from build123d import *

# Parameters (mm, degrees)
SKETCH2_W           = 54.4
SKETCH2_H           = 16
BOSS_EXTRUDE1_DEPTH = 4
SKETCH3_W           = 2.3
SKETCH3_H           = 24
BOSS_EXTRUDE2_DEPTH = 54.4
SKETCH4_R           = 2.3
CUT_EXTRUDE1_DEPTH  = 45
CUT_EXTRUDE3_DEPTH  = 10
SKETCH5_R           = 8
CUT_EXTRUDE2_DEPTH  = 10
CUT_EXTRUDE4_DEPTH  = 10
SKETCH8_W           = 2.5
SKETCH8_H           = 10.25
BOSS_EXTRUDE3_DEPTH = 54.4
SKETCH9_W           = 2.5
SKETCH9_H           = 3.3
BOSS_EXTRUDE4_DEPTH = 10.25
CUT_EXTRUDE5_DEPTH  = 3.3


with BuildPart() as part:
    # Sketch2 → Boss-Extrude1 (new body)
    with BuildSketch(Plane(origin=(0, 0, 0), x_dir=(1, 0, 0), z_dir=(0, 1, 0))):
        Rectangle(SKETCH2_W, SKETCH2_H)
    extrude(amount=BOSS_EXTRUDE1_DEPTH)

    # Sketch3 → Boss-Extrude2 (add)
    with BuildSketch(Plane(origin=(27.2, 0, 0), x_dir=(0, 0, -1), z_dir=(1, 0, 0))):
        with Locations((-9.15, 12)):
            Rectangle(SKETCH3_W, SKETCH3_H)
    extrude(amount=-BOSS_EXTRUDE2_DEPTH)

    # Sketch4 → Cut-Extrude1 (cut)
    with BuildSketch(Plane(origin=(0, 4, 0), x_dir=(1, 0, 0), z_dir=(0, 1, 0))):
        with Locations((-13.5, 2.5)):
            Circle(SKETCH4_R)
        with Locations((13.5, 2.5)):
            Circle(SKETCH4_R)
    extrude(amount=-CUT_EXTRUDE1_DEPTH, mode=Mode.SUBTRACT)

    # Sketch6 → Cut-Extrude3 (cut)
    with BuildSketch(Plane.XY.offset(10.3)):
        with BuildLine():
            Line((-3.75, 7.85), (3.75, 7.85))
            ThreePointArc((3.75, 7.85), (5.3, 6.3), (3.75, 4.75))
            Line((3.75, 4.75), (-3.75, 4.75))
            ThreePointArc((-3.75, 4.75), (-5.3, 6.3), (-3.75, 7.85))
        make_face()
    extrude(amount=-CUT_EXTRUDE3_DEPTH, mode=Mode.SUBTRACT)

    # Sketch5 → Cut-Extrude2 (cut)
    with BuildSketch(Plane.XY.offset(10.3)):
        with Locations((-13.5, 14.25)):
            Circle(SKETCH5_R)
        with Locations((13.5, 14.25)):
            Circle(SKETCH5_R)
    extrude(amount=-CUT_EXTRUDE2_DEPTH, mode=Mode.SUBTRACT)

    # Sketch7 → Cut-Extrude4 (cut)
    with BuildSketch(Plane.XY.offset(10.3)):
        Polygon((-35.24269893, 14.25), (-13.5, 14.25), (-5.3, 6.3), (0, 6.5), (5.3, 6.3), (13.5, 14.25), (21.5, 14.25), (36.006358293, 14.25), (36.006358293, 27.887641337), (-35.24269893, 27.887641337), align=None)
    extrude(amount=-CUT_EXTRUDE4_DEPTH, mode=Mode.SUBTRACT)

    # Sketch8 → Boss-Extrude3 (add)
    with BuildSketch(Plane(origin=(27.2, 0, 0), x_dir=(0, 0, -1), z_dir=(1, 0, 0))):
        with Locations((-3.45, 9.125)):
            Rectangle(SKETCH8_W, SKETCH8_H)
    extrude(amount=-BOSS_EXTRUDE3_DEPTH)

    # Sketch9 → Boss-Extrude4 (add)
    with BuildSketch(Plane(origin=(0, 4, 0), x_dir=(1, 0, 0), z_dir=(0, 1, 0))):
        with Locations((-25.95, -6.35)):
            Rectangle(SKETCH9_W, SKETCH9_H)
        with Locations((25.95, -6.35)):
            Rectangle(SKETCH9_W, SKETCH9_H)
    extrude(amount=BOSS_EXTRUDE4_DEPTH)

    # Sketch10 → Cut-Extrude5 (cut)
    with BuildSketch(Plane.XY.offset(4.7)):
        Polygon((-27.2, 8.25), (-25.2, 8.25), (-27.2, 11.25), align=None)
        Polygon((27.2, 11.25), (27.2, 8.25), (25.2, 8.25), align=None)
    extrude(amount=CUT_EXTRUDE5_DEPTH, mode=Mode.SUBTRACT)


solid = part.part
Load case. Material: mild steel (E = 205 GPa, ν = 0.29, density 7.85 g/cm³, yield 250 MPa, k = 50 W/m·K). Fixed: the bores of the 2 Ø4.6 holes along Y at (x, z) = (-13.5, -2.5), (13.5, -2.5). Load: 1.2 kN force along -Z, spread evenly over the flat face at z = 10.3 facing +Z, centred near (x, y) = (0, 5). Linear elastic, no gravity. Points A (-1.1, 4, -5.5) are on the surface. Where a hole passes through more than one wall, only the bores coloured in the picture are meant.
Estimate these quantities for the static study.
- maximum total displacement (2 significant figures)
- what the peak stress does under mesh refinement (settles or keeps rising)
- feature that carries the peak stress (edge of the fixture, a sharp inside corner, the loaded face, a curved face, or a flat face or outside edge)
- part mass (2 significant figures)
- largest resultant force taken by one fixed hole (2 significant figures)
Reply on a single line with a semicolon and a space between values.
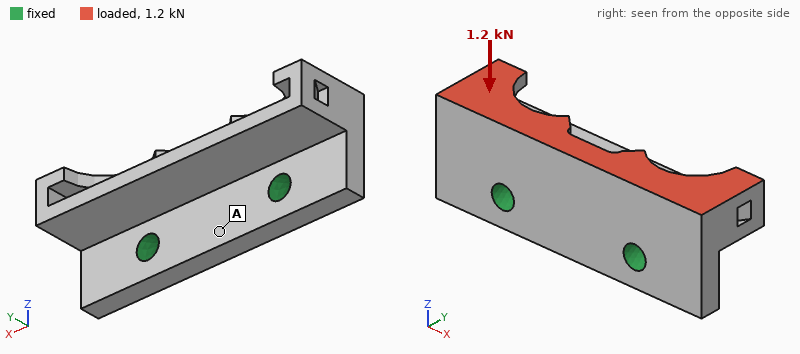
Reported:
12 µm; keeps rising; edge of the fixture; 47 g; 610 N
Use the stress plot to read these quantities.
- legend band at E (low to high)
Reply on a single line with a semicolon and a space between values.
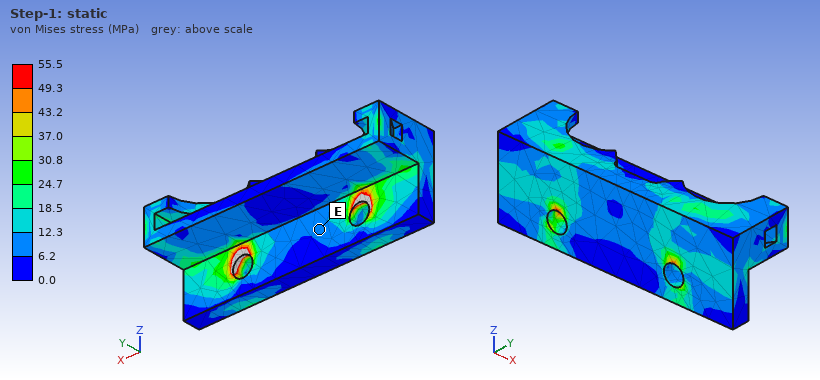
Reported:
6.2 to 12.3 MPa
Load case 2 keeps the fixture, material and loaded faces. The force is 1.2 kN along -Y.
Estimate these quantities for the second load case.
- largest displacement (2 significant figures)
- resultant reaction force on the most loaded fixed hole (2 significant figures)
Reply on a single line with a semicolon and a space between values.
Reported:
28 µm; 610 N
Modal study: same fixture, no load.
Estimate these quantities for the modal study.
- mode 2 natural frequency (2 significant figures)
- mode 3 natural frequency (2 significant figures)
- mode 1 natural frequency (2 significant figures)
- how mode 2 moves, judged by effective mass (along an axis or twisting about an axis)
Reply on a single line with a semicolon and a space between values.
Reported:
10 kHz; 17 kHz; 9400 Hz; twisting about Z
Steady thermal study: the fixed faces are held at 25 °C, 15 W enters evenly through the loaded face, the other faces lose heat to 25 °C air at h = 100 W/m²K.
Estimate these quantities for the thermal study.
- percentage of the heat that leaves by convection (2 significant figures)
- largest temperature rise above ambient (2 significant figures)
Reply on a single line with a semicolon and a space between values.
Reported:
24 %; 21 K
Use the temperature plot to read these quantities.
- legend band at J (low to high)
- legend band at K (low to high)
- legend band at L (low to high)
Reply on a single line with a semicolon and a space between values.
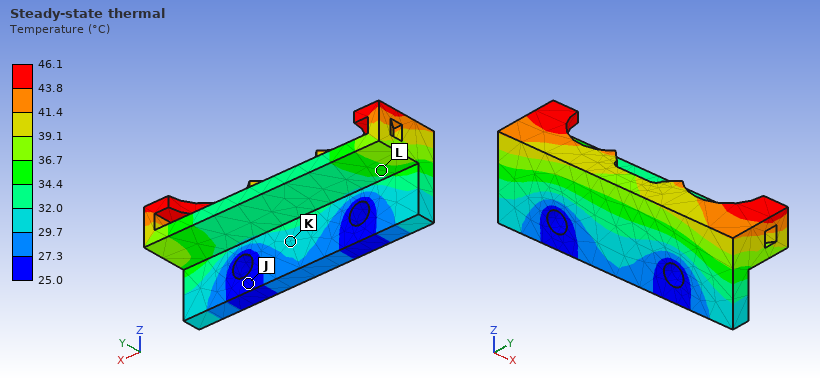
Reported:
25.0 to 27.3 °C; 29.7 to 32.0 °C; 34.4 to 36.7 °C
